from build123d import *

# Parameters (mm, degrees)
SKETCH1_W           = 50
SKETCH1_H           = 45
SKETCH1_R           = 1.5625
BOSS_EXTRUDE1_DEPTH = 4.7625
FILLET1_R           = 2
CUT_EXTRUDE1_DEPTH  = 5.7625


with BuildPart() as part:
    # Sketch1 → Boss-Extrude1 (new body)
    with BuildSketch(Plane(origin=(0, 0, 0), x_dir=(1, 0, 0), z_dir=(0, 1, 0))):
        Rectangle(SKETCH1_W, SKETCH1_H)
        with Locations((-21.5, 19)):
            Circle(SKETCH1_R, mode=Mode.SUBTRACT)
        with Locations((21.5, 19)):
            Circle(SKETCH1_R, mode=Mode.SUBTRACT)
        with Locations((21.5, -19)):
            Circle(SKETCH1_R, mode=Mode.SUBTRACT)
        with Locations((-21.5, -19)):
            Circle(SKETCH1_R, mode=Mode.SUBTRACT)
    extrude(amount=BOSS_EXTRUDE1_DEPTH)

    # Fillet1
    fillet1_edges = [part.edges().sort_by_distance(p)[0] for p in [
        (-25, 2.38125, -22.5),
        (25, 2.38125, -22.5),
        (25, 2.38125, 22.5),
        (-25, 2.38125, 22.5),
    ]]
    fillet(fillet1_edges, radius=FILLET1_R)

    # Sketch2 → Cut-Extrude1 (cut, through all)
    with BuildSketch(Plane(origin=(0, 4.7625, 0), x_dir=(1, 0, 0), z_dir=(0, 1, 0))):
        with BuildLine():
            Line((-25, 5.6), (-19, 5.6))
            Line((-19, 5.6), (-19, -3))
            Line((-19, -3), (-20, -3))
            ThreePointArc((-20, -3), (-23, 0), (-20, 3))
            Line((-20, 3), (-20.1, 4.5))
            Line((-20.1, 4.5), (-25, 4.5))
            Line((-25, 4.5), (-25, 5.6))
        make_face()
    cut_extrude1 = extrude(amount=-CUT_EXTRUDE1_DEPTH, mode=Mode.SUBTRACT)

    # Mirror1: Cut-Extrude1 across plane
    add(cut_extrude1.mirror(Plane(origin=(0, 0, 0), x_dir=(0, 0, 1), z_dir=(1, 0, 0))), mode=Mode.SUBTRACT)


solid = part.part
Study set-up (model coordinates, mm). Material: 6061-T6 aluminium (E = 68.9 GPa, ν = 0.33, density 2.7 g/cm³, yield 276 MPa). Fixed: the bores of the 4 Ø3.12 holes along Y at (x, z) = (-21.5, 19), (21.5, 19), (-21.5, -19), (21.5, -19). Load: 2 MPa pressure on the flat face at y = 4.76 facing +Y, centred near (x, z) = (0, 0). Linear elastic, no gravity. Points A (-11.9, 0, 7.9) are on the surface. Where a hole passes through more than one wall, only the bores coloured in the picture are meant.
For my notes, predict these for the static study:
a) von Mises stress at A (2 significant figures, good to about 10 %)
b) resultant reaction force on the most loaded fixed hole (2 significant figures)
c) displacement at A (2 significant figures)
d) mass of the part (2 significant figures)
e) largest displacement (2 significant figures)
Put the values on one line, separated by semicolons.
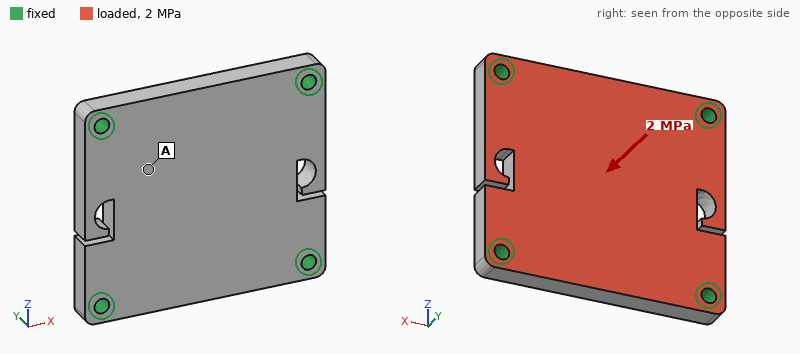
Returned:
32 MPa; 1.1 kN; 49 µm; 28 g; 70 µm
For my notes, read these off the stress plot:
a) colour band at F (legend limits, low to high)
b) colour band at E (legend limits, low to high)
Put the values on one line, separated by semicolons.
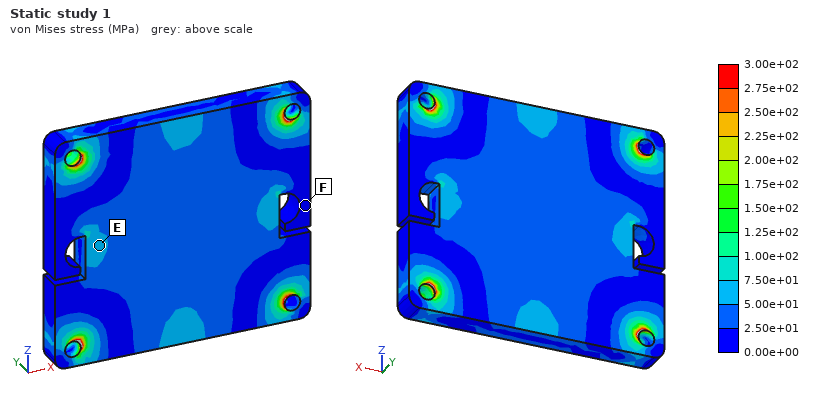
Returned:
0.00e+00 to 2.50e+01 MPa; 5.00e+01 to 7.50e+01 MPa
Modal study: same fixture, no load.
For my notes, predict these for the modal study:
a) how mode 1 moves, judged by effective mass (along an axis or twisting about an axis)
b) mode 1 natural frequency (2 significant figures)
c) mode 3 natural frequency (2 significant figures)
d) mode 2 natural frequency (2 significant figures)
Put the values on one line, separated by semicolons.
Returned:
along Y; 8900 Hz; 14 kHz; 14 kHz
